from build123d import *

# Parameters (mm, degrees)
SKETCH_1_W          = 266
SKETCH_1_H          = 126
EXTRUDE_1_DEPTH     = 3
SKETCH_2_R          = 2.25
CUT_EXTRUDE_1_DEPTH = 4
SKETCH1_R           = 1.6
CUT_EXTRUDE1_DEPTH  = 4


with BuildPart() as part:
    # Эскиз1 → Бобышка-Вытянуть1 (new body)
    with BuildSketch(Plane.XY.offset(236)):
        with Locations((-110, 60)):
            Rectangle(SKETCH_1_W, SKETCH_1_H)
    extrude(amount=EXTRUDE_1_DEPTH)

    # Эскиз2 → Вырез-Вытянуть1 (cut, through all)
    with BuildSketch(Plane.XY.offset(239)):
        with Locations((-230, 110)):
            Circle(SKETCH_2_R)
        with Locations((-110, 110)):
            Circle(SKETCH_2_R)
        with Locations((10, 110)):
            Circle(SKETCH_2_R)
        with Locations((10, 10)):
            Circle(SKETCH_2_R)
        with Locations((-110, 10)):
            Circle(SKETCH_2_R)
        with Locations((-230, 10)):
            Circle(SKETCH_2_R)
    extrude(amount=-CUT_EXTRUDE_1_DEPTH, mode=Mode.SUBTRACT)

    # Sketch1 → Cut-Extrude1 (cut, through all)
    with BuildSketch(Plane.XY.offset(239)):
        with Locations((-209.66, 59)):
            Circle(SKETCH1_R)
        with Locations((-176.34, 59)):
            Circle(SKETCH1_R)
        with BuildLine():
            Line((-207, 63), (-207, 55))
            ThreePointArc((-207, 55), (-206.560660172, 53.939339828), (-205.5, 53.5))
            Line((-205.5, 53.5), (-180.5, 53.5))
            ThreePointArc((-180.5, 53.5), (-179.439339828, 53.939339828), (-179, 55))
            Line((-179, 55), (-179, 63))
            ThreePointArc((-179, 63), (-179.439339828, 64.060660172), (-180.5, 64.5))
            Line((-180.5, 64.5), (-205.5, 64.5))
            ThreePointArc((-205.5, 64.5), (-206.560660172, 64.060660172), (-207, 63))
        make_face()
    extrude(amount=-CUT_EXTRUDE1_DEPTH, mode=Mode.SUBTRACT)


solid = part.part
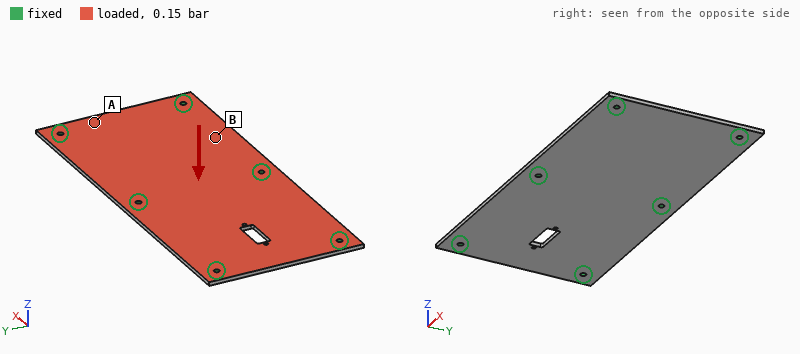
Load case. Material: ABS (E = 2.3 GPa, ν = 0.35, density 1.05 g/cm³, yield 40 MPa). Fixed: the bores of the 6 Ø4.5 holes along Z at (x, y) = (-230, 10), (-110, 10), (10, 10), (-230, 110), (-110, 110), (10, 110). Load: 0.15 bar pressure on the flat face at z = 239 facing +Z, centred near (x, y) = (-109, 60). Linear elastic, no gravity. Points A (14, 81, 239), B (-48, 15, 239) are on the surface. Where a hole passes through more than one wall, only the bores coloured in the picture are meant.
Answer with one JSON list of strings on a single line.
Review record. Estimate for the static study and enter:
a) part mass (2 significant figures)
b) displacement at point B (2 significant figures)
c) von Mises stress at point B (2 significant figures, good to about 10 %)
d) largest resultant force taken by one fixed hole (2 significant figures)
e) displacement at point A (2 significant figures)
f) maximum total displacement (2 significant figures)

["100 g", "2.0 mm", "6.5 MPa", "120 N", "0.67 mm", "3.0 mm"]
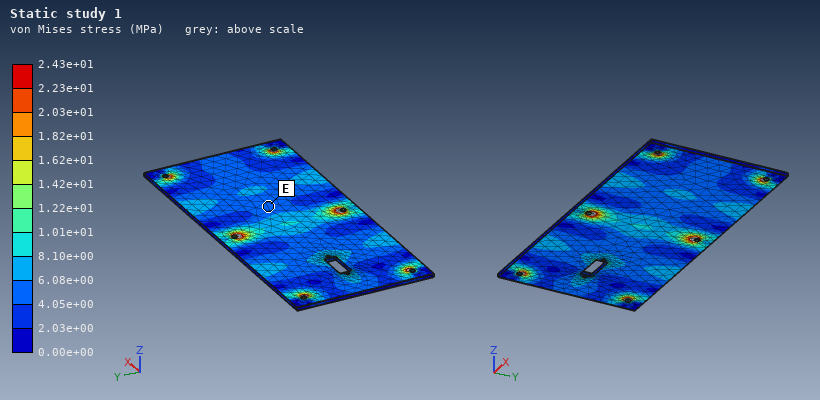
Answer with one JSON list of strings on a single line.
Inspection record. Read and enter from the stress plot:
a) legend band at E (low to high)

["4.05e+00 to 6.08e+00 MPa"]
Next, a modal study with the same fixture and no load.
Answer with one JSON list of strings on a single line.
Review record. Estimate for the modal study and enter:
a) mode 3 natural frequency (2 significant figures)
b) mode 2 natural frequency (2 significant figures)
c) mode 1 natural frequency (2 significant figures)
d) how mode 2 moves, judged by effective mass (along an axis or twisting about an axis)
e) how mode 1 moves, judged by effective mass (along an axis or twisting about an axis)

["360 Hz", "250 Hz", "240 Hz", "along Z", "twisting about Y"]
